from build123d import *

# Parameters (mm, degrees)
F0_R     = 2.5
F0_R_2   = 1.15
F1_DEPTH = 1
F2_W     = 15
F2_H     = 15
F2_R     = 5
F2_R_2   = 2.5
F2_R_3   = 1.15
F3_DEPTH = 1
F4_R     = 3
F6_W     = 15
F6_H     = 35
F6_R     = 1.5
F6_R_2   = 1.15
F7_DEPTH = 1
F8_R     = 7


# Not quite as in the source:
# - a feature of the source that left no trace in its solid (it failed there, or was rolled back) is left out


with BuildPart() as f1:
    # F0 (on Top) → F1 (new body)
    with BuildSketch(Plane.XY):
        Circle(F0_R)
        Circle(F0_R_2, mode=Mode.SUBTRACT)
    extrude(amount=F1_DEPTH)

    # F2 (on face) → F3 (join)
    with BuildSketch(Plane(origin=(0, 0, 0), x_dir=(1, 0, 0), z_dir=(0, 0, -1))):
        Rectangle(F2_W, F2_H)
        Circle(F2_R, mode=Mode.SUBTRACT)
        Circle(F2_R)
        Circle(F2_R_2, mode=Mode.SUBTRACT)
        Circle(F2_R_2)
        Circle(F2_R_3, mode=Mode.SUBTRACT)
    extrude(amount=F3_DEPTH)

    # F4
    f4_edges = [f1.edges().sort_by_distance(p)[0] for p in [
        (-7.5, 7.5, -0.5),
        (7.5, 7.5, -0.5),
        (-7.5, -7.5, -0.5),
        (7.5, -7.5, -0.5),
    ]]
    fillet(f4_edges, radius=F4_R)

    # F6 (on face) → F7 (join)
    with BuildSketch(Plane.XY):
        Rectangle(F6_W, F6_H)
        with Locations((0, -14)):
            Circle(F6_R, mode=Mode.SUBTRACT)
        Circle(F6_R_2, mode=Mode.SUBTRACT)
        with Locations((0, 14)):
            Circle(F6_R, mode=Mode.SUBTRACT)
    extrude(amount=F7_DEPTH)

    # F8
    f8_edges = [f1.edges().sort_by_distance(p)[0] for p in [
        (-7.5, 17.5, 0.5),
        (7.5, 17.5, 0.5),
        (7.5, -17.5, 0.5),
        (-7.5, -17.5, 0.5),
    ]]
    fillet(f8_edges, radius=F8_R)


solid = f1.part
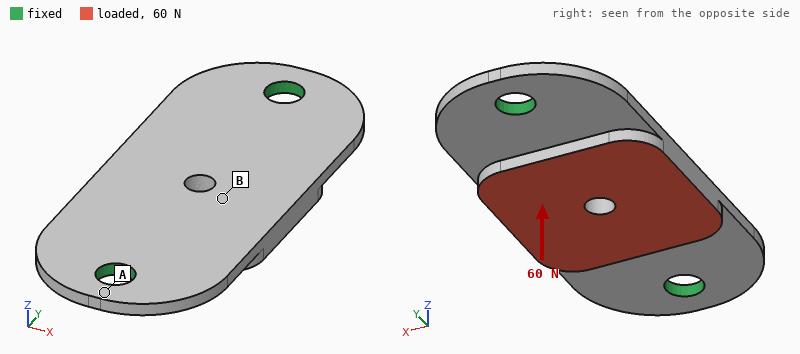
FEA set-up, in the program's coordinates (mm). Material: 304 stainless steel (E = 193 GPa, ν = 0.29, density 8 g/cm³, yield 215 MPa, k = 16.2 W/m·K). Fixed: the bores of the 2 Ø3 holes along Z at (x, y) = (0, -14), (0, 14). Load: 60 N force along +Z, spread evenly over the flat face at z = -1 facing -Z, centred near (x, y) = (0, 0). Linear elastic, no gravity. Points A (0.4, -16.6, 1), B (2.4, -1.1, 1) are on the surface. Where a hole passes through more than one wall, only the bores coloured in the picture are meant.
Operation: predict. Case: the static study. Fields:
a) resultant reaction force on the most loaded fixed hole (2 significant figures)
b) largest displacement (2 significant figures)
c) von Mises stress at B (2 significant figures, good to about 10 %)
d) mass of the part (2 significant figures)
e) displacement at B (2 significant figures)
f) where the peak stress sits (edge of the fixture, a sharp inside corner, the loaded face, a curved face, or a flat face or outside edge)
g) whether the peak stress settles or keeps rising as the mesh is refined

60 N
7.9 µm
16 MPa
5.4 g
7.2 µm
edge of the fixture
keeps rising
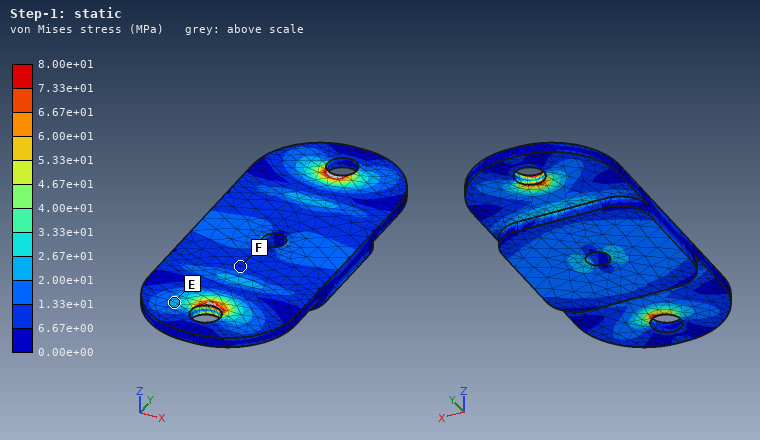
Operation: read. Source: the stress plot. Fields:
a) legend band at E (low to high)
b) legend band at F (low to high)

2.00e+01 to 2.67e+01 MPa
6.67e+00 to 1.33e+01 MPa
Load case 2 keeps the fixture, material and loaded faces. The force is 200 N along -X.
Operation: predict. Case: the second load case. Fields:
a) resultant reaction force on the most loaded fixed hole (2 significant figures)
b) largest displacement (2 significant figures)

100 N
17 µm
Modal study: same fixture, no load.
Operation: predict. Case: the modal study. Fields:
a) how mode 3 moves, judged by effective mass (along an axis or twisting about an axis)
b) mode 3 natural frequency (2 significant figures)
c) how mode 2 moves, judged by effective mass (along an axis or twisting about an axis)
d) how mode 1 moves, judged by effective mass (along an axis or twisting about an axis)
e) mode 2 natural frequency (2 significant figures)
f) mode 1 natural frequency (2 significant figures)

twisting about X
18 kHz
along Z
twisting about Y
7700 Hz
6900 Hz
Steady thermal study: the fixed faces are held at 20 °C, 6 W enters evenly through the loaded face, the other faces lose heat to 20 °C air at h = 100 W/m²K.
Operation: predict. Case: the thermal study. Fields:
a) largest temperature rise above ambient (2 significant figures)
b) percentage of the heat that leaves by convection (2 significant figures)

70 K
54 %
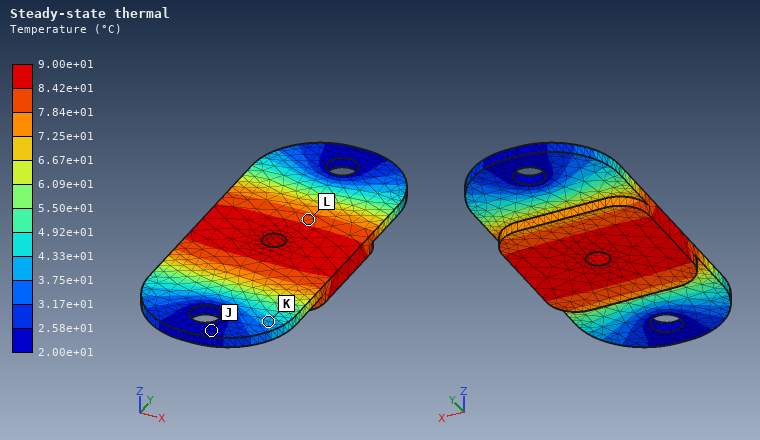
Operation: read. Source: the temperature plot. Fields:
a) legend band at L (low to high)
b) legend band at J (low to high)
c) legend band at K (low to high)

7.84e+01 to 8.42e+01 °C
2.00e+01 to 2.58e+01 °C
3.75e+01 to 4.33e+01 °C
